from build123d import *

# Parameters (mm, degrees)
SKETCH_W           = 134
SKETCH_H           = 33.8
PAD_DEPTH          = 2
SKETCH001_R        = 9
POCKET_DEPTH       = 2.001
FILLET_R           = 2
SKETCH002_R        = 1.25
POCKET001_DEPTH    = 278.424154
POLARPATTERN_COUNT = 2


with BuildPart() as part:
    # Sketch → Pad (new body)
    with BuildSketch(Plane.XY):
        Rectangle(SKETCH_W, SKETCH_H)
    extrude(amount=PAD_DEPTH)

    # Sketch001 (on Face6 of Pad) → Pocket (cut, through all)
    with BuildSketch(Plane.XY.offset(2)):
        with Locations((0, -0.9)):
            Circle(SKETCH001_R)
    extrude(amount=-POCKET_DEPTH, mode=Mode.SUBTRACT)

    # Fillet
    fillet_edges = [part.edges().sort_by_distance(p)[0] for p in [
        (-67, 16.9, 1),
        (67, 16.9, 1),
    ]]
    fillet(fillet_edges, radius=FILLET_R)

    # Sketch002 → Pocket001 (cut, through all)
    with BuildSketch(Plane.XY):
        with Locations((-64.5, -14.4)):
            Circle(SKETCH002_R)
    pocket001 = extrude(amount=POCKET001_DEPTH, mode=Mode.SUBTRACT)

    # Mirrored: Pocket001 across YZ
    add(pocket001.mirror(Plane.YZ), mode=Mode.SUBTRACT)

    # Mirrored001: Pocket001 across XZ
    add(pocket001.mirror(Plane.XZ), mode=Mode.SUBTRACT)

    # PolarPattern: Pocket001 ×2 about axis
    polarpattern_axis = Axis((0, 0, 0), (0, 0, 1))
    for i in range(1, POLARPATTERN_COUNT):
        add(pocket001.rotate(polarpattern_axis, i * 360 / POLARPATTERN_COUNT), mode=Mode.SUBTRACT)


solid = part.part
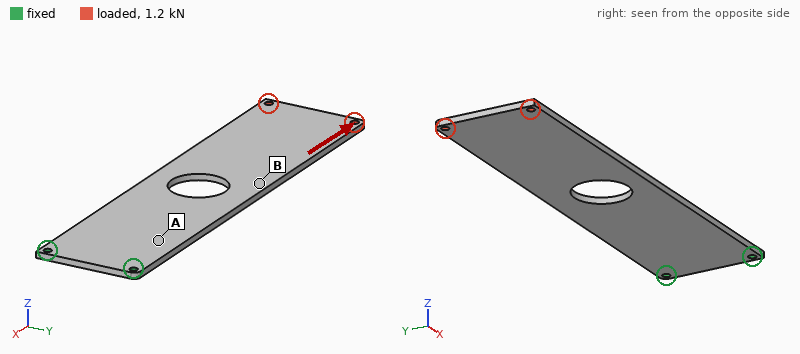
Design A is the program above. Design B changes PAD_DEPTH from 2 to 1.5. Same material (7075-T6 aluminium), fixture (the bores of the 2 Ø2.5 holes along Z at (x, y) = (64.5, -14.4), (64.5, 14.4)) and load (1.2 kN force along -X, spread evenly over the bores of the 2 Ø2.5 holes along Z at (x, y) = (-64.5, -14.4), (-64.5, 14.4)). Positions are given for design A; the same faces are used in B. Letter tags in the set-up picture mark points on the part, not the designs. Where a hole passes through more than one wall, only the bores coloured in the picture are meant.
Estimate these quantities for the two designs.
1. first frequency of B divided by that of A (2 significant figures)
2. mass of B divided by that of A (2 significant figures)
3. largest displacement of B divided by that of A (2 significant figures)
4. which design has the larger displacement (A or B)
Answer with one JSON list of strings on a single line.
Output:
["0.75", "0.75", "1.3", "B"]
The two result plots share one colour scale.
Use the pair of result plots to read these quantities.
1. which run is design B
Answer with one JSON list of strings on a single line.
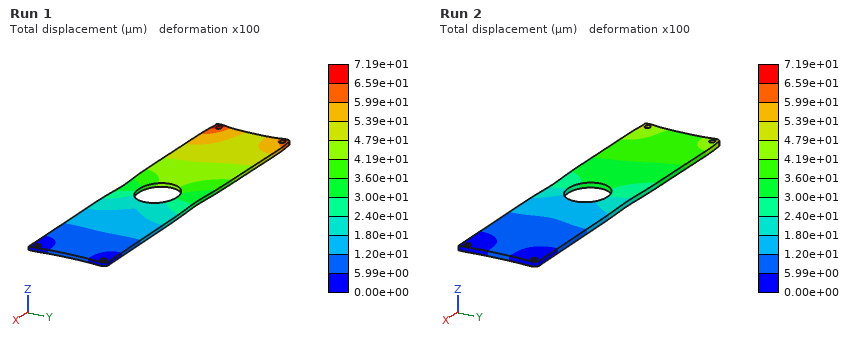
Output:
["Run 1"]
